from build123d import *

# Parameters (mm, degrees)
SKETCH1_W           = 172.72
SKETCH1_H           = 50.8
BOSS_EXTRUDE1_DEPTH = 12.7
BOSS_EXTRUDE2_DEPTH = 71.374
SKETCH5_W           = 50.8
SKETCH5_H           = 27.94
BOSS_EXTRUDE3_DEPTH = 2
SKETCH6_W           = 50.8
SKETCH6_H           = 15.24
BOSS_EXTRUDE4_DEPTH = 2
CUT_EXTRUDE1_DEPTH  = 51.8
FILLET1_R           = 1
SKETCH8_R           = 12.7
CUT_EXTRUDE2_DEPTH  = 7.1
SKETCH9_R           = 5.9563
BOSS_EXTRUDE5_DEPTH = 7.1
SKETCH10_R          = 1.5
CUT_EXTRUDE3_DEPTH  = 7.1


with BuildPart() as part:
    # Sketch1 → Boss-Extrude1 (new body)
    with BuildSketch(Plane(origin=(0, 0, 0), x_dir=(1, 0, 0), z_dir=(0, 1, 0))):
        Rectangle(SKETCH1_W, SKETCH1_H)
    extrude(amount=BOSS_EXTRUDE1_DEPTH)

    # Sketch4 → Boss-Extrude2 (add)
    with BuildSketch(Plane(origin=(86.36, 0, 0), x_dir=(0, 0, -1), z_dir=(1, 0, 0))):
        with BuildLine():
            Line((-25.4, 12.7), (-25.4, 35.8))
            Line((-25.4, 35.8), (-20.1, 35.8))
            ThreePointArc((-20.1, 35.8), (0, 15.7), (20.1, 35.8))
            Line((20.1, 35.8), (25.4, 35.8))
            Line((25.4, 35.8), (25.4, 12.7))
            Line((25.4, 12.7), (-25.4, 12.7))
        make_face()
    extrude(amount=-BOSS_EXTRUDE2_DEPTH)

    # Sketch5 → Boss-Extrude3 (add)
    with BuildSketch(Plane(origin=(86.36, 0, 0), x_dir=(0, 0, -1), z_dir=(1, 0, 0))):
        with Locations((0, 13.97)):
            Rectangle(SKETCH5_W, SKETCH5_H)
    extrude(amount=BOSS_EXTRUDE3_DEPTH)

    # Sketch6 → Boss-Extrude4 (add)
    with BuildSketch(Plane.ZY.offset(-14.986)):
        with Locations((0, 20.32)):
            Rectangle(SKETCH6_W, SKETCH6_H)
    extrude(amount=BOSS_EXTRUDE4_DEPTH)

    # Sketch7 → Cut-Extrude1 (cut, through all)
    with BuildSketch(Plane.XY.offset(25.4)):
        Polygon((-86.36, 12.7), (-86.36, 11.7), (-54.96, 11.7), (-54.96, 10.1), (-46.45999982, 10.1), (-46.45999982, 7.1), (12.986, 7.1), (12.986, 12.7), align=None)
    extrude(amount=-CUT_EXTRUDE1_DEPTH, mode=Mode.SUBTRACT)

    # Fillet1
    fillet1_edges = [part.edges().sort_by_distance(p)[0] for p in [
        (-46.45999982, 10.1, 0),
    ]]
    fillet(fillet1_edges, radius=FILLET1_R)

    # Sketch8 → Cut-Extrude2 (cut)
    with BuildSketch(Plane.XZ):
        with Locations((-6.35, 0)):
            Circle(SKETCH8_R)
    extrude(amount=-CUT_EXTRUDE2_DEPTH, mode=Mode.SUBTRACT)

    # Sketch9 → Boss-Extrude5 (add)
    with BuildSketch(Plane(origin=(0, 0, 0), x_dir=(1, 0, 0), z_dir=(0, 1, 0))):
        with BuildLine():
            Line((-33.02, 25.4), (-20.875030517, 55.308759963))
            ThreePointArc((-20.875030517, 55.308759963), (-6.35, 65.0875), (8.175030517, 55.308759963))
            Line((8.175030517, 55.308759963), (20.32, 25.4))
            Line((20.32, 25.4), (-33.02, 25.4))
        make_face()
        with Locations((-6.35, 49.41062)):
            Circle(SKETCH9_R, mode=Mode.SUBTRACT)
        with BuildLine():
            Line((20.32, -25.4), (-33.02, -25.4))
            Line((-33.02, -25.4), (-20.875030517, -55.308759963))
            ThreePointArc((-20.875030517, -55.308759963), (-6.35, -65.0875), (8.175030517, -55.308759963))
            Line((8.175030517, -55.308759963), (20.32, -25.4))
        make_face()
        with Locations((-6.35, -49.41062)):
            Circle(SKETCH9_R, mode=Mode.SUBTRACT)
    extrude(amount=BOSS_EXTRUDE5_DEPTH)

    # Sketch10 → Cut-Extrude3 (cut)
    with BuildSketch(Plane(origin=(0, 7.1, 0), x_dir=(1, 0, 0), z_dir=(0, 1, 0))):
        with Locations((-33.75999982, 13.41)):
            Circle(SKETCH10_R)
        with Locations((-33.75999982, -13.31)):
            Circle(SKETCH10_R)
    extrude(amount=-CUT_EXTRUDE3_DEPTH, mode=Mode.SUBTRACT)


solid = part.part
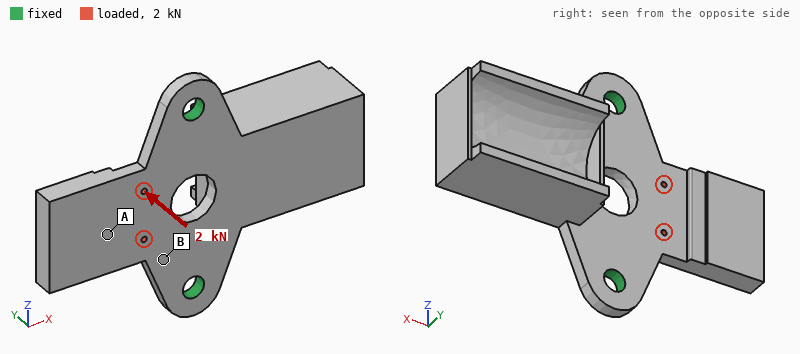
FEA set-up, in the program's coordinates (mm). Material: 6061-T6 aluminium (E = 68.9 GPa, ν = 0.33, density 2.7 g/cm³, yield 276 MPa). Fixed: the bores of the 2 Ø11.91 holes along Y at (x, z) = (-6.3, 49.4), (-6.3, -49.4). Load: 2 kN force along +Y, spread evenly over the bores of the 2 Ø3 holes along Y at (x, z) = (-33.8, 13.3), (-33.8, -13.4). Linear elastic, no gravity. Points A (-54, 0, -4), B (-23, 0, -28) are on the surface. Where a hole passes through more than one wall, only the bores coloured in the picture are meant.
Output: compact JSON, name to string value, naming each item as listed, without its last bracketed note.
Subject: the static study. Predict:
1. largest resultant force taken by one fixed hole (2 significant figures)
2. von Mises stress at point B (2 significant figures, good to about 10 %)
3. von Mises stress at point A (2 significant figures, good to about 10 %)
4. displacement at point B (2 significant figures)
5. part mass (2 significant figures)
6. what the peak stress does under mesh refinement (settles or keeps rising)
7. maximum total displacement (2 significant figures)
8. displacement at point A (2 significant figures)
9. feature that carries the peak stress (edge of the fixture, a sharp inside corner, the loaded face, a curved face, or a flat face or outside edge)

{"largest resultant force taken by one fixed hole": "1.0 kN", "von Mises stress at point B": "64 MPa", "von Mises stress at point A": "14 MPa", "displacement at point B": "0.10 mm", "part mass": "400 g", "what the peak stress does under mesh refinement": "keeps rising", "maximum total displacement": "0.67 mm", "displacement at point A": "0.40 mm", "feature that carries the peak stress": "edge of the fixture"}
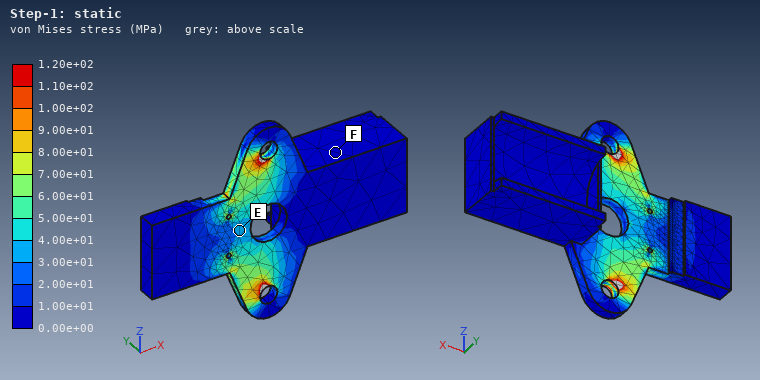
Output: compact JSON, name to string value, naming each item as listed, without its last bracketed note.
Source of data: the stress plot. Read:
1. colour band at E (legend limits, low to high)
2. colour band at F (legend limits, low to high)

{"colour band at E": "3.00e+01 to 4.00e+01 MPa", "colour band at F": "0.00e+00 to 1.00e+01 MPa"}
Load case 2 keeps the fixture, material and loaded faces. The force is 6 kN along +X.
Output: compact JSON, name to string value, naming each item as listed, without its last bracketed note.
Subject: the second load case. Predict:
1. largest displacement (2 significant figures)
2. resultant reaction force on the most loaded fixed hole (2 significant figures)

{"largest displacement": "23 µm", "resultant reaction force on the most loaded fixed hole": "3.1 kN"}
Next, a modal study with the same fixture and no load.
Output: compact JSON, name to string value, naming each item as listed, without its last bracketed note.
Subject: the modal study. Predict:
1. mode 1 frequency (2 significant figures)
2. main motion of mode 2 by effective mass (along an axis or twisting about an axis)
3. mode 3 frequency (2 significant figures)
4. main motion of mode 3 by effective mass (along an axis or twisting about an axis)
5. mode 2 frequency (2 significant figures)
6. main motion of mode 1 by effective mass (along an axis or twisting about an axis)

{"mode 1 frequency": "410 Hz", "main motion of mode 2 by effective mass": "along Y", "mode 3 frequency": "2500 Hz", "main motion of mode 3 by effective mass": "along Z", "mode 2 frequency": "710 Hz", "main motion of mode 1 by effective mass": "along Y"}
